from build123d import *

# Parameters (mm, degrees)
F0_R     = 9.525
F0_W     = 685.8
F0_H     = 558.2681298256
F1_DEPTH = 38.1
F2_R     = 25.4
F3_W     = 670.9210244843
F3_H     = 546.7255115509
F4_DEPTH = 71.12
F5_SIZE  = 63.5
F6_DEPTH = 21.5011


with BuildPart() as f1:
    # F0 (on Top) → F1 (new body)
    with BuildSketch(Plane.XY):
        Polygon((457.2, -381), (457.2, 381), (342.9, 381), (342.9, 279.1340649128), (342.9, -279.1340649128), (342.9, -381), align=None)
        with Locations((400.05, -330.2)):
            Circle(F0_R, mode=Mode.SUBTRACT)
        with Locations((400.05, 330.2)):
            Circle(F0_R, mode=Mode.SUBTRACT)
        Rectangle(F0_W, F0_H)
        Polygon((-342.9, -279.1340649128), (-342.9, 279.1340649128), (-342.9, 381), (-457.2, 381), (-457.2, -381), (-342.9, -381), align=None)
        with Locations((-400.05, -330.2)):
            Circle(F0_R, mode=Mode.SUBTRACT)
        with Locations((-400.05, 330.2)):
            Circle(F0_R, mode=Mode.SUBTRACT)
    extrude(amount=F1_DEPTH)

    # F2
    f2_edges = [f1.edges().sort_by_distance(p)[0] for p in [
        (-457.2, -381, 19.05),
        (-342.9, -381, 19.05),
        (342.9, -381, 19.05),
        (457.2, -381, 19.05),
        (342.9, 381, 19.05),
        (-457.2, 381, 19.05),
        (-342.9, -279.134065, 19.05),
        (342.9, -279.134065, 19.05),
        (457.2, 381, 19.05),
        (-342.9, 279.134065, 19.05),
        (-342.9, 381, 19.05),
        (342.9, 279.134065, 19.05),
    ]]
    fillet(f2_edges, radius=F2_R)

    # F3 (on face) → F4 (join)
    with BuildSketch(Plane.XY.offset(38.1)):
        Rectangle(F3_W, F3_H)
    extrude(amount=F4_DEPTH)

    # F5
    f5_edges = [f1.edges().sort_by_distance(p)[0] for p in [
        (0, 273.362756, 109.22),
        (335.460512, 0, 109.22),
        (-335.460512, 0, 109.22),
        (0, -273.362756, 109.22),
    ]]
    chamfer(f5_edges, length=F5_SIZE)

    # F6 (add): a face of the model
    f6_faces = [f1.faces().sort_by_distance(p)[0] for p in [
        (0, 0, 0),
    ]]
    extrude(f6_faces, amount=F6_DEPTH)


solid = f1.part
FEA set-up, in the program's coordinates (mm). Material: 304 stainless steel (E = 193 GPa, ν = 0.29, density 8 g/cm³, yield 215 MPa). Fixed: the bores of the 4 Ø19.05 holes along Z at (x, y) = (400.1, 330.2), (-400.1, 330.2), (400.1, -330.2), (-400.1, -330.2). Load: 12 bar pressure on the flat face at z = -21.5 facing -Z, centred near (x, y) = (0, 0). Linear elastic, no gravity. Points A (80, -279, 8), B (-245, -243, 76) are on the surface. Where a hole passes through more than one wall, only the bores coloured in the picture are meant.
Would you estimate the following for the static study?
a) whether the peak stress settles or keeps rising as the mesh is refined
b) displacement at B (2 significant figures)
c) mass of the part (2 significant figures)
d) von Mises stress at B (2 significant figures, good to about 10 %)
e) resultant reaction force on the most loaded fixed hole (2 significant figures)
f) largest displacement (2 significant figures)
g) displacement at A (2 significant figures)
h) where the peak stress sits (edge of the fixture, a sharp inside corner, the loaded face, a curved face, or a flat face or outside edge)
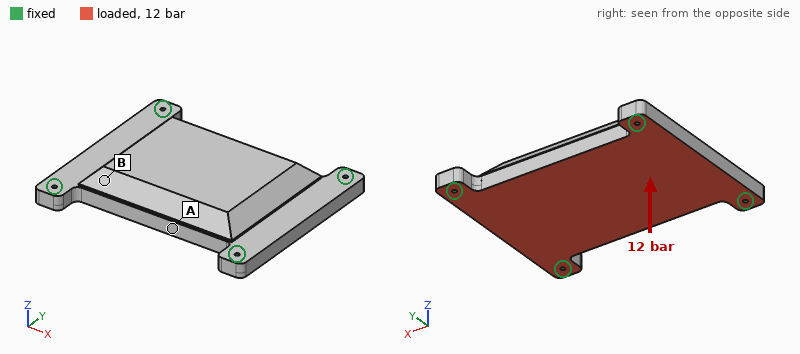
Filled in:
keeps rising
0.24 mm
440 kg
43 MPa
190 kN
0.32 mm
0.31 mm
edge of the fixture
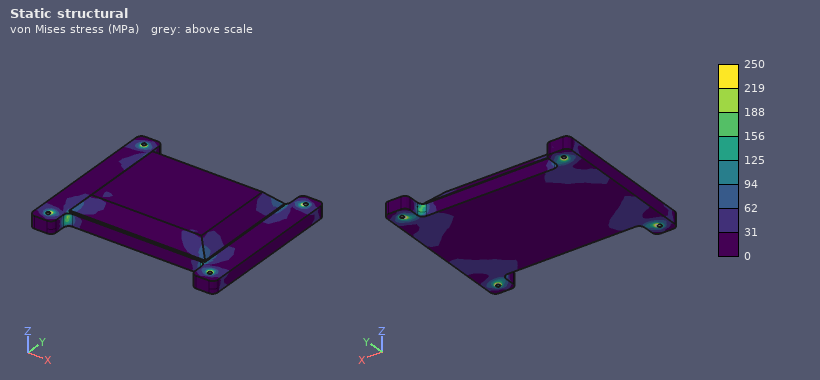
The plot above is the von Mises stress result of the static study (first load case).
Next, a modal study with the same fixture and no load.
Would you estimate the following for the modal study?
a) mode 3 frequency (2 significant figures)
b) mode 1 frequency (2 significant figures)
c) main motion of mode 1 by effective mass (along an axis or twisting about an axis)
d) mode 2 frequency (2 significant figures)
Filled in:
680 Hz
350 Hz
along Z
650 Hz
